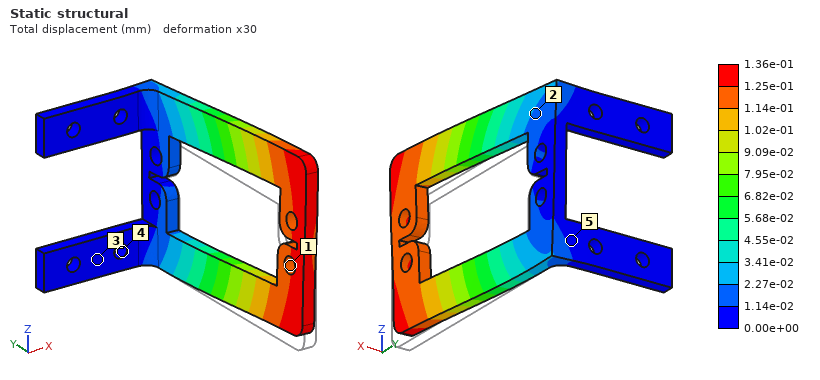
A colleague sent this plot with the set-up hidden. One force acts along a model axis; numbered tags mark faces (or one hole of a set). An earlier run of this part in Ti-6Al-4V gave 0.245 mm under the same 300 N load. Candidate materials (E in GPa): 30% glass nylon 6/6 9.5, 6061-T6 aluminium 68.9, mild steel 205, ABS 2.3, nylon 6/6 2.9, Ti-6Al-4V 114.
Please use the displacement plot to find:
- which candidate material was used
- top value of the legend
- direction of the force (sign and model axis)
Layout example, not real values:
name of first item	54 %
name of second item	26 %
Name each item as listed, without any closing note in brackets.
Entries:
which candidate material was used	mild steel
top value of the legend	1.36e-01 mm
direction of the force	+Z
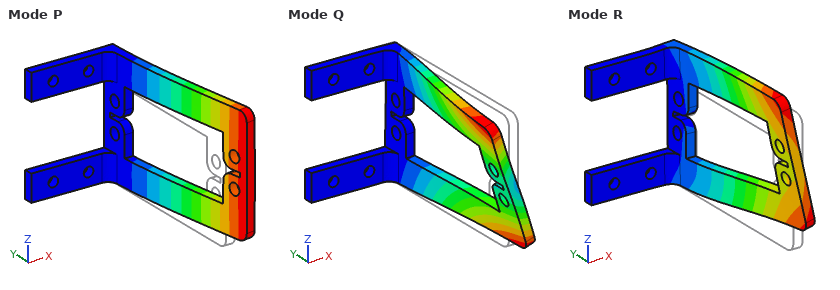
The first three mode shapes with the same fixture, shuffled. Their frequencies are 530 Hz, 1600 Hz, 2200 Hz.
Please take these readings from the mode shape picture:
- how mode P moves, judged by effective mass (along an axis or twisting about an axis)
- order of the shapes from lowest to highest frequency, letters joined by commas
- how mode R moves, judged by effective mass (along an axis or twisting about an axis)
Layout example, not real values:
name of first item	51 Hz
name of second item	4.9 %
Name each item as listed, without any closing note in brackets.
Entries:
how mode P moves, judged by effective mass	along X
order of the shapes from lowest to highest frequency, letters joined by commas	P, Q, R
how mode R moves, judged by effective mass	along Z
